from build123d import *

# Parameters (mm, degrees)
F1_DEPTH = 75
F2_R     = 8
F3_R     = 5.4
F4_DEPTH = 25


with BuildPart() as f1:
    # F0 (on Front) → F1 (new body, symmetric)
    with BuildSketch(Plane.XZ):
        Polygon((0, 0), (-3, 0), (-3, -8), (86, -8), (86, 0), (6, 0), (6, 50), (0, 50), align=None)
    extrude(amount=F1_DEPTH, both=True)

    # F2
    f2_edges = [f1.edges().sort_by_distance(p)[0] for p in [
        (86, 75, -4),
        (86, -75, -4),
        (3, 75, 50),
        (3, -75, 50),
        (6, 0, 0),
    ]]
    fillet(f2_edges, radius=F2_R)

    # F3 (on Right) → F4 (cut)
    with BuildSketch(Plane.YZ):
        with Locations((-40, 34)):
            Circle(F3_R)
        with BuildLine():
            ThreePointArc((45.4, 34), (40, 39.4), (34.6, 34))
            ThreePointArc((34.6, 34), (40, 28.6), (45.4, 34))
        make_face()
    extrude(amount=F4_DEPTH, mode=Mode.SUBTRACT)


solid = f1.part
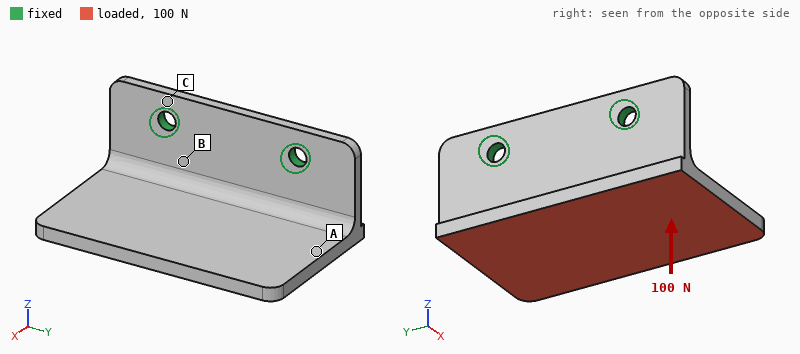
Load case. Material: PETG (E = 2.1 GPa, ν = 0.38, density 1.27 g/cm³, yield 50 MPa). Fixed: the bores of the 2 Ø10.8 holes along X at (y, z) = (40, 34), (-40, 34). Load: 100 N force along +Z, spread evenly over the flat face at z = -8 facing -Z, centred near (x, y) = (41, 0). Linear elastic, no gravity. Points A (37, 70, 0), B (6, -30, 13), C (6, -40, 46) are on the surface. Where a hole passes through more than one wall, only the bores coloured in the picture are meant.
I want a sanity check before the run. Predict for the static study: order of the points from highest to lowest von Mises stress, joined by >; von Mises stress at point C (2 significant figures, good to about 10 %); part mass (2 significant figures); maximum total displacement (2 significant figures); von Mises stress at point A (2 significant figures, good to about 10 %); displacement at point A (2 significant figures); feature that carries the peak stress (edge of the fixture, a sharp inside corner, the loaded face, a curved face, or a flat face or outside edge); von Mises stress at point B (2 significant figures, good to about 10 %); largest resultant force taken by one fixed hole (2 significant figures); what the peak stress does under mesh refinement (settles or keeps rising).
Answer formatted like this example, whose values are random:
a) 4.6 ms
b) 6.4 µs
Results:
a) B > C > A
b) 2.0 MPa
c) 190 g
d) 2.2 mm
e) 0.78 MPa
f) 0.87 mm
g) edge of the fixture
h) 4.2 MPa
i) 51 N
j) keeps rising
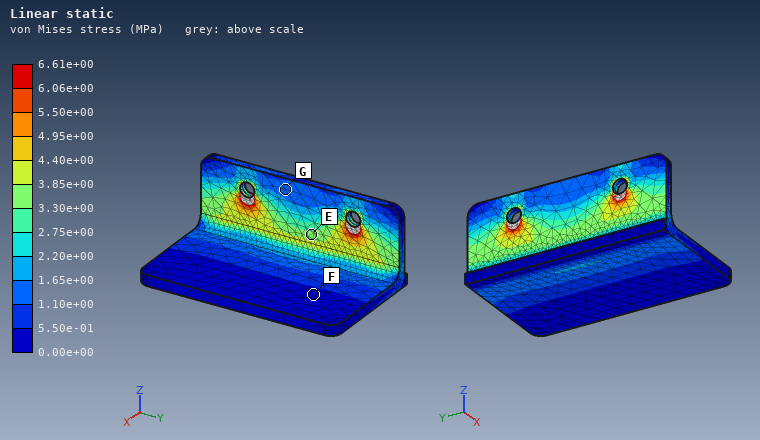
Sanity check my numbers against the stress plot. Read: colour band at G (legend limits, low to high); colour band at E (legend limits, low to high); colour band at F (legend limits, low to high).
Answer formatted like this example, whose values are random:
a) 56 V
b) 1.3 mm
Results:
a) 1.10e+00 to 1.65e+00 MPa
b) 3.30e+00 to 3.85e+00 MPa
c) 0.00e+00 to 5.50e-01 MPa
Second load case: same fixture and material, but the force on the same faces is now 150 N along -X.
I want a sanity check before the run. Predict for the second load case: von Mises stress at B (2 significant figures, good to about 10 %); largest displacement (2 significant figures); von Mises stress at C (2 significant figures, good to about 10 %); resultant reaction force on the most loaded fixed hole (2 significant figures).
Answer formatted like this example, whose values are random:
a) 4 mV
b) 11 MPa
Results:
a) 3.4 MPa
b) 2.0 mm
c) 2.3 MPa
d) 75 N
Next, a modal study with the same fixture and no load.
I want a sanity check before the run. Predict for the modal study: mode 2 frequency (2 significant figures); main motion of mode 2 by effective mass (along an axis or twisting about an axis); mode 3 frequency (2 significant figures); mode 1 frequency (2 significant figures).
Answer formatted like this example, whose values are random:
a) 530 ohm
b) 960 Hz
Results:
a) 230 Hz
b) along Y
c) 390 Hz
d) 110 Hz
